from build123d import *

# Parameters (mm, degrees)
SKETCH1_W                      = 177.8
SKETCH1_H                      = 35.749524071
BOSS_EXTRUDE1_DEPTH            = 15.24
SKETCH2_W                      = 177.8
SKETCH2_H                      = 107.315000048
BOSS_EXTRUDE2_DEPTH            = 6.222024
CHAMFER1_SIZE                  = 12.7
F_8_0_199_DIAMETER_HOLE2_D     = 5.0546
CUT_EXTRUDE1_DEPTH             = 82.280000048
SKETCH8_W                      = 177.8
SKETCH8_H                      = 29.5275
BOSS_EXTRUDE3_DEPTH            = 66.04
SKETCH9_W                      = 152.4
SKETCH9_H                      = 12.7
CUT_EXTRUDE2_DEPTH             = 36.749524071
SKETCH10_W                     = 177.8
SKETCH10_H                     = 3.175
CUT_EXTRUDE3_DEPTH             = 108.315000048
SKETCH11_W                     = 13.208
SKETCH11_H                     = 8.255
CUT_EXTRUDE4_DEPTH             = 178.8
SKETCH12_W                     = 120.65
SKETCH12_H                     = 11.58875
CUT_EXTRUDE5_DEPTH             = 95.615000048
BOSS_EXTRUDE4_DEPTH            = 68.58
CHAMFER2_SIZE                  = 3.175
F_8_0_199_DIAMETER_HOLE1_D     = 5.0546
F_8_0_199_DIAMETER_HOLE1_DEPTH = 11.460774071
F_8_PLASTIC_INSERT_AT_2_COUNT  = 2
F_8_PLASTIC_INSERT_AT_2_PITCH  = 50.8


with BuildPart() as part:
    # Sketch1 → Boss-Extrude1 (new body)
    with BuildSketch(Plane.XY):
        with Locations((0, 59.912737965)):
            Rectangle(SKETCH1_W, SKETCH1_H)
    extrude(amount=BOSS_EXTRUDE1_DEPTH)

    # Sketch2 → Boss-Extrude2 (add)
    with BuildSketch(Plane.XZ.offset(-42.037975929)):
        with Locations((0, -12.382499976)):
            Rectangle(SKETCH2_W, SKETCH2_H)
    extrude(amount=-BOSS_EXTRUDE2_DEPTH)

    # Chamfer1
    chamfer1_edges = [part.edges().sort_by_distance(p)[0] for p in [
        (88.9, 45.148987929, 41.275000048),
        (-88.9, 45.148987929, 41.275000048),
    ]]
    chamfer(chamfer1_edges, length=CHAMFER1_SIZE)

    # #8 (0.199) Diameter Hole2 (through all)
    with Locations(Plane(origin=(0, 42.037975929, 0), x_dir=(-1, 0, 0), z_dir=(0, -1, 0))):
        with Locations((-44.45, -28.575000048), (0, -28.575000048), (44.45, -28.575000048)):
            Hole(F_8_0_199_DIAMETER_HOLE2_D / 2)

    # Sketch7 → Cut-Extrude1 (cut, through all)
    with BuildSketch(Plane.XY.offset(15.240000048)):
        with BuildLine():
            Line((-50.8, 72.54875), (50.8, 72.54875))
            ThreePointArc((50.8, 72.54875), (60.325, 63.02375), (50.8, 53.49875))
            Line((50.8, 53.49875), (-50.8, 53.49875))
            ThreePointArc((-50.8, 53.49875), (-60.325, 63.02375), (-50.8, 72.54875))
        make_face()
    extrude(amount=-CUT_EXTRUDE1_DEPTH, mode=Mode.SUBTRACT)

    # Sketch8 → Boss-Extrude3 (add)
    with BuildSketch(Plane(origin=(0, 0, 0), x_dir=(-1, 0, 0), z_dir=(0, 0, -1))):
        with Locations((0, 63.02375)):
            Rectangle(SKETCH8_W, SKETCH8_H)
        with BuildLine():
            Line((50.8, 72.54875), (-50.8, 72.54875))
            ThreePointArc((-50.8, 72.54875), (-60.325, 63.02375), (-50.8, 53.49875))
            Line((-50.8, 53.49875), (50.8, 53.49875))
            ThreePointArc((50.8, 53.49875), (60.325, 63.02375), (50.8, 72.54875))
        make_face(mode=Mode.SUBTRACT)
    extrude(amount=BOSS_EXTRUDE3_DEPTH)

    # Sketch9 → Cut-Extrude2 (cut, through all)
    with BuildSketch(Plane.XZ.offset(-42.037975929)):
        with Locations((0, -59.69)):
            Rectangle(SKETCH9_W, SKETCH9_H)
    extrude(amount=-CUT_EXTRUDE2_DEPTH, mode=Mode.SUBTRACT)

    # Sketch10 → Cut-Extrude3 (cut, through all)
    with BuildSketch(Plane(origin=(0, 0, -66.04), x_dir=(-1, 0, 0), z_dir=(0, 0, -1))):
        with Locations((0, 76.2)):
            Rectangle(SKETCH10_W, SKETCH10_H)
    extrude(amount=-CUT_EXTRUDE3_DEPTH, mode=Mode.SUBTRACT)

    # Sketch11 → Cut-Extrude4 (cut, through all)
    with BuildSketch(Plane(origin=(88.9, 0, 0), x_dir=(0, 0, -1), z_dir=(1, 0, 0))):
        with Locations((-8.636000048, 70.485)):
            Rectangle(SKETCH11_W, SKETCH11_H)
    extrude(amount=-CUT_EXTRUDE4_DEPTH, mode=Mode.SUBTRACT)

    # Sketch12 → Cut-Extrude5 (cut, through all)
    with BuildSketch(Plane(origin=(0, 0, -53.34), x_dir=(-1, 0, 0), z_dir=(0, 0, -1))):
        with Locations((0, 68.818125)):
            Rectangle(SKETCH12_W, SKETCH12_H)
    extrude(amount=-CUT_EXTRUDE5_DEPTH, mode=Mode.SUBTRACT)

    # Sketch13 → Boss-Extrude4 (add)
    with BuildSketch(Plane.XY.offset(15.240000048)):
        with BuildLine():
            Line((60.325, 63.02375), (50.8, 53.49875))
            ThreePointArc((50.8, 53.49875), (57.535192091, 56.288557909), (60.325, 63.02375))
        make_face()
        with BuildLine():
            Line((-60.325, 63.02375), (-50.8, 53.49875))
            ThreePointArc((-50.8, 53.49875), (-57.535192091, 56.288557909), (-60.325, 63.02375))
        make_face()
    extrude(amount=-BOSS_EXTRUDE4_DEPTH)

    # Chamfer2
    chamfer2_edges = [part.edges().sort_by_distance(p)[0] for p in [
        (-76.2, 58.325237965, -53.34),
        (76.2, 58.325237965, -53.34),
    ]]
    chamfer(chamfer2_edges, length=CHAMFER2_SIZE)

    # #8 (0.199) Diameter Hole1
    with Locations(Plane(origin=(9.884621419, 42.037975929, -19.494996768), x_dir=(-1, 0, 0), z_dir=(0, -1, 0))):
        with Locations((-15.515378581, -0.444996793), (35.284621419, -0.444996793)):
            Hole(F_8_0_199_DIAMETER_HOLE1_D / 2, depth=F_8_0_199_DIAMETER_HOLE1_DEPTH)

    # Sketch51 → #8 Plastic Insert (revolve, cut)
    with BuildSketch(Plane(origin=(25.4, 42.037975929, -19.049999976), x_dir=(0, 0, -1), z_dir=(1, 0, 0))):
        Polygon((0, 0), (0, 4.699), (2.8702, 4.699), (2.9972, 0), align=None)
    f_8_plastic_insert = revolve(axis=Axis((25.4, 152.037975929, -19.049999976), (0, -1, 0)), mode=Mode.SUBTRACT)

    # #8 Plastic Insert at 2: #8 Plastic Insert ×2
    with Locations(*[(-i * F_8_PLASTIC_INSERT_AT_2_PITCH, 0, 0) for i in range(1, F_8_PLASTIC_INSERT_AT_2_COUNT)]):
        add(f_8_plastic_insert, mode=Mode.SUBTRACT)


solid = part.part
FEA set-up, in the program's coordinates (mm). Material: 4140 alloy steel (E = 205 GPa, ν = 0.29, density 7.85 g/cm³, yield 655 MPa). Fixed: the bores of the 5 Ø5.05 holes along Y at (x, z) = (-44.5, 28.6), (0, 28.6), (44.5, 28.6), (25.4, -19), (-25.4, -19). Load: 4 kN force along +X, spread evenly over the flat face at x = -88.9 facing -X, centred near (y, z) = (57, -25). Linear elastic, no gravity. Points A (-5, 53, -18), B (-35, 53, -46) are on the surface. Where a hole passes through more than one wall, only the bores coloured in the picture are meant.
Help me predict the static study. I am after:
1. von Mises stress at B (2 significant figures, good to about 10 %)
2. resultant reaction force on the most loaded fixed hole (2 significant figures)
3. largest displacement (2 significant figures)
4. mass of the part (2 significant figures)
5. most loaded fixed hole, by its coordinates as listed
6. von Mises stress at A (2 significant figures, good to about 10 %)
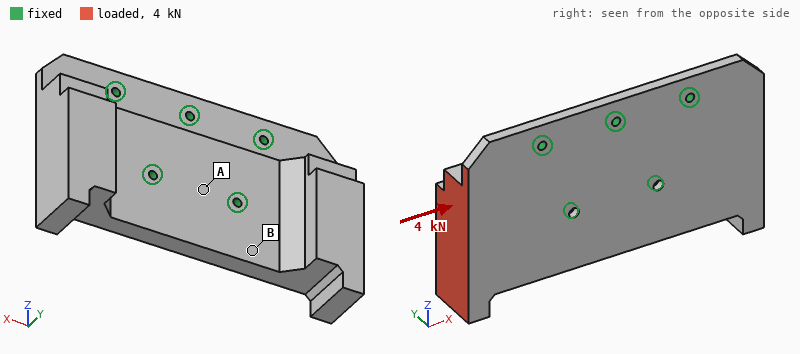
21 MPa
3.1 kN
43 µm
2.0 kg
(-25.4, -19)
3.6 MPa
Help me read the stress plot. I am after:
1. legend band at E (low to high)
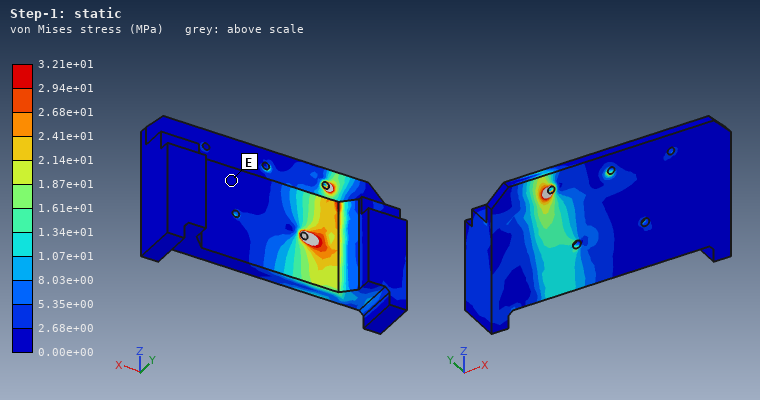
0.00e+00 to 2.68e+00 MPa
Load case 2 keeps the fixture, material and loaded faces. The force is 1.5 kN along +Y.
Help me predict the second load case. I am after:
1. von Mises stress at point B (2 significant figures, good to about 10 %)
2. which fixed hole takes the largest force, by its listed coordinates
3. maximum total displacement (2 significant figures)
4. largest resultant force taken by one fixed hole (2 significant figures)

29 MPa
(-25.4, -19)
98 µm
3.0 kN
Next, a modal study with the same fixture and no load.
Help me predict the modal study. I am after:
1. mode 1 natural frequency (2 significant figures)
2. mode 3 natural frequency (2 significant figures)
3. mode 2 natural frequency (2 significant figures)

1200 Hz
3300 Hz
1200 Hz
